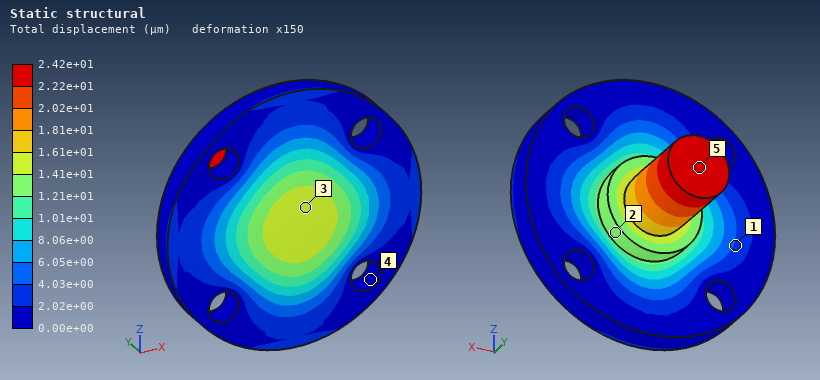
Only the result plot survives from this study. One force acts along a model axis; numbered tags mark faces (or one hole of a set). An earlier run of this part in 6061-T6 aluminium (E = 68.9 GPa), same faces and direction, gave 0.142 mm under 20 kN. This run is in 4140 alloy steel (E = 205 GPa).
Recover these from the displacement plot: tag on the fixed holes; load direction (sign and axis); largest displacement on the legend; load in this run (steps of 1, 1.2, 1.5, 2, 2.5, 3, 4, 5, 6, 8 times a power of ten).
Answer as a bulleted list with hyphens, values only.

- 4
- -Y
- 2.42e+01 µm
- 10 kN
